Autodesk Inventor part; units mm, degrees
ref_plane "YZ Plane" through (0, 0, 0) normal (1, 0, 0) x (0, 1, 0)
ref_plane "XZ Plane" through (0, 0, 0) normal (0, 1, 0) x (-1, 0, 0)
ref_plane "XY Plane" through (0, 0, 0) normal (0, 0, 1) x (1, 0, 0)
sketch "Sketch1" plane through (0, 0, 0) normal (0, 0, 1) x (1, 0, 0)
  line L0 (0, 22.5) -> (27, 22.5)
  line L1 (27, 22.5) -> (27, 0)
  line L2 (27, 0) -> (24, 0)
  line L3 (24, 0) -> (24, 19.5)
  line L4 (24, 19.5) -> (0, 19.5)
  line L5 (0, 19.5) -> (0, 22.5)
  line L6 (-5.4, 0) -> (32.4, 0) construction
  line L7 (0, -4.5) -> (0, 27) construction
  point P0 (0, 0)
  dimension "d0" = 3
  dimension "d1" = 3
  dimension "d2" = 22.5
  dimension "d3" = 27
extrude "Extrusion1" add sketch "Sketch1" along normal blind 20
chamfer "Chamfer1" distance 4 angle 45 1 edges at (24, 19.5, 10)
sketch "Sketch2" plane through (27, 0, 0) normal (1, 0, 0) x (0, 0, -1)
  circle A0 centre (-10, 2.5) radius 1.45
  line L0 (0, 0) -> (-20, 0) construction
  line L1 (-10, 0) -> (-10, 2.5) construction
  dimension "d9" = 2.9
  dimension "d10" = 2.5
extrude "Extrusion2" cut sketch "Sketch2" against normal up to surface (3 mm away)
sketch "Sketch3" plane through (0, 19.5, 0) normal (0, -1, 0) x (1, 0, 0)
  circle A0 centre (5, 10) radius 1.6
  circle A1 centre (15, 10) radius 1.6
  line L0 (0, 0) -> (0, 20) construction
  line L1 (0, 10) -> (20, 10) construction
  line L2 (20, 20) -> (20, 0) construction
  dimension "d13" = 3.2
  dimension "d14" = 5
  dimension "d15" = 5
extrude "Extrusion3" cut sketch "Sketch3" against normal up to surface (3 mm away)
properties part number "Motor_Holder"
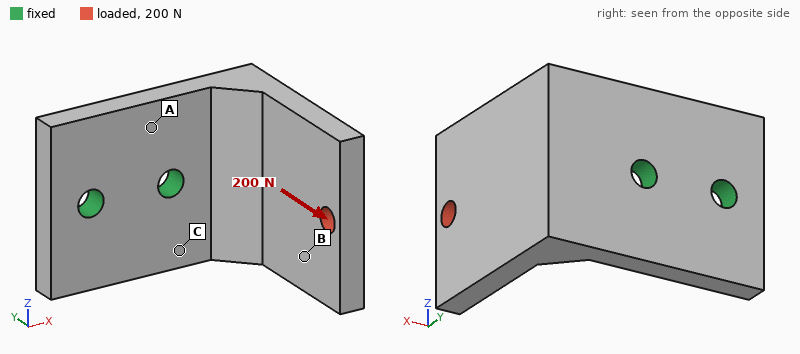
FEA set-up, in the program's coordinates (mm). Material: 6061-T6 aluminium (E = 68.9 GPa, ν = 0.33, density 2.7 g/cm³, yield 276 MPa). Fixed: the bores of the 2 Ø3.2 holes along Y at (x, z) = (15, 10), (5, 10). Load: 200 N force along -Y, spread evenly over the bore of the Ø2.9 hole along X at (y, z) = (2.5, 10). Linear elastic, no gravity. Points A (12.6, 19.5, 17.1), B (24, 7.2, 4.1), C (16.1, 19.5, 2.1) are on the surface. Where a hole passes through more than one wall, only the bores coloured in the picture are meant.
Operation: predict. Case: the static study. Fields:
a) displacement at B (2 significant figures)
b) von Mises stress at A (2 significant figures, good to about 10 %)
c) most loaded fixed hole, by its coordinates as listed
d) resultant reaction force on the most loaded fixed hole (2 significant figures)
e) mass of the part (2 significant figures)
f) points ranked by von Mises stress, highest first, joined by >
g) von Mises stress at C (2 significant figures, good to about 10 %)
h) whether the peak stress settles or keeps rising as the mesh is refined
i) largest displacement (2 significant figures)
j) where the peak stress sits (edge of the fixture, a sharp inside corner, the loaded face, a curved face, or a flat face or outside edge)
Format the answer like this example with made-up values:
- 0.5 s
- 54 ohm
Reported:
- 49 µm
- 19 MPa
- (15, 10)
- 270 N
- 7.8 g
- C > A > B
- 32 MPa
- keeps rising
- 75 µm
- edge of the fixture
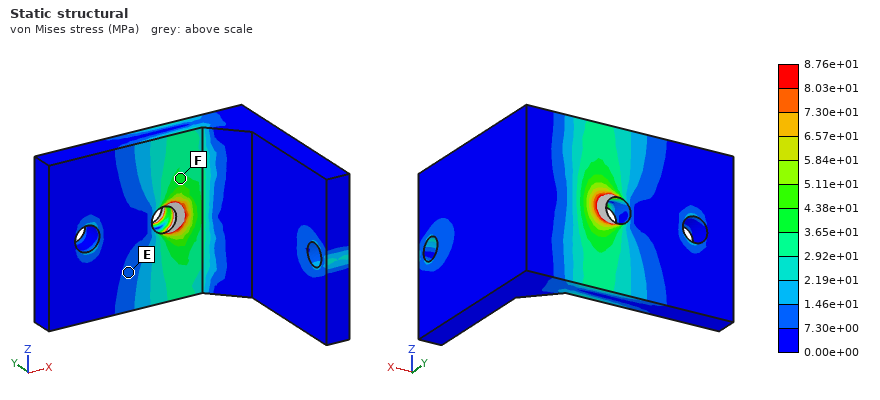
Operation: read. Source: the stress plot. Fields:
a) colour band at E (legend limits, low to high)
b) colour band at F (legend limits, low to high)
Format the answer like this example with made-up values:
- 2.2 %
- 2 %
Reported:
- 7.30e+00 to 1.46e+01 MPa
- 3.65e+01 to 4.38e+01 MPa
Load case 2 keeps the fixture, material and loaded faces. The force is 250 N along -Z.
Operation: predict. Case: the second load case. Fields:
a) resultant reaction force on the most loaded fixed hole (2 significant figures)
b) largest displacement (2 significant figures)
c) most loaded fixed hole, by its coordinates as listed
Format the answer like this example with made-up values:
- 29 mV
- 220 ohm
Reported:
- 420 N
- 0.15 mm
- (15, 10)
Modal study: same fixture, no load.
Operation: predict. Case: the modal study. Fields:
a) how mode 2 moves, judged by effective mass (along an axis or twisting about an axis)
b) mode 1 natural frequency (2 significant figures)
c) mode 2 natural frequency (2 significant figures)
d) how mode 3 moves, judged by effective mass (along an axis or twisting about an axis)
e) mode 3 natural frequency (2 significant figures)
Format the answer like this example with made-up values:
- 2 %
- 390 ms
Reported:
- along Z
- 3800 Hz
- 5300 Hz
- along Y
- 12 kHz
